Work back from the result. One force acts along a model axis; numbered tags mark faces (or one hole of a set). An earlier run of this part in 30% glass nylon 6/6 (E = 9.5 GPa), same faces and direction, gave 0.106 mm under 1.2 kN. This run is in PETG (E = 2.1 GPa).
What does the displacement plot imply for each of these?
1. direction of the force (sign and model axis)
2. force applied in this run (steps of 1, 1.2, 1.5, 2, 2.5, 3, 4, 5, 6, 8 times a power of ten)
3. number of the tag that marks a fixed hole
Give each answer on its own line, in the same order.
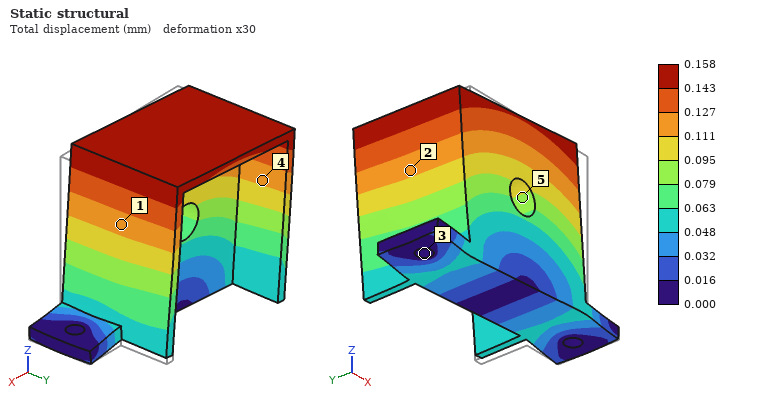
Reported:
-X
400 N
3
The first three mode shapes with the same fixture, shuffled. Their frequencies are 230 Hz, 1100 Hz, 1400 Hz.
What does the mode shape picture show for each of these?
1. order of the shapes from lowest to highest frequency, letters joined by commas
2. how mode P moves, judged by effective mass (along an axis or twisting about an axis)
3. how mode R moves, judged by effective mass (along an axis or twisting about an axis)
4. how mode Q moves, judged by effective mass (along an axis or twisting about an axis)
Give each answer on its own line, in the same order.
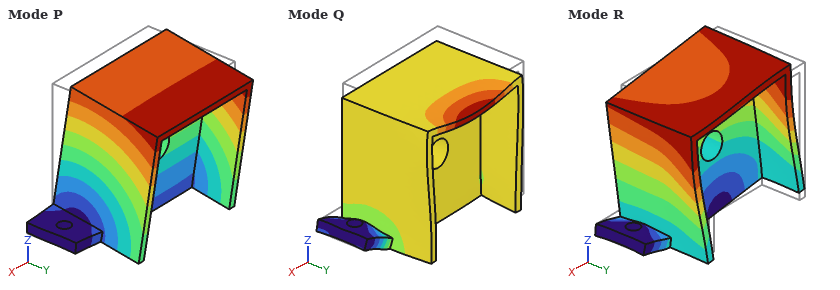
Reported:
P, R, Q
along Y
along X
along Z
